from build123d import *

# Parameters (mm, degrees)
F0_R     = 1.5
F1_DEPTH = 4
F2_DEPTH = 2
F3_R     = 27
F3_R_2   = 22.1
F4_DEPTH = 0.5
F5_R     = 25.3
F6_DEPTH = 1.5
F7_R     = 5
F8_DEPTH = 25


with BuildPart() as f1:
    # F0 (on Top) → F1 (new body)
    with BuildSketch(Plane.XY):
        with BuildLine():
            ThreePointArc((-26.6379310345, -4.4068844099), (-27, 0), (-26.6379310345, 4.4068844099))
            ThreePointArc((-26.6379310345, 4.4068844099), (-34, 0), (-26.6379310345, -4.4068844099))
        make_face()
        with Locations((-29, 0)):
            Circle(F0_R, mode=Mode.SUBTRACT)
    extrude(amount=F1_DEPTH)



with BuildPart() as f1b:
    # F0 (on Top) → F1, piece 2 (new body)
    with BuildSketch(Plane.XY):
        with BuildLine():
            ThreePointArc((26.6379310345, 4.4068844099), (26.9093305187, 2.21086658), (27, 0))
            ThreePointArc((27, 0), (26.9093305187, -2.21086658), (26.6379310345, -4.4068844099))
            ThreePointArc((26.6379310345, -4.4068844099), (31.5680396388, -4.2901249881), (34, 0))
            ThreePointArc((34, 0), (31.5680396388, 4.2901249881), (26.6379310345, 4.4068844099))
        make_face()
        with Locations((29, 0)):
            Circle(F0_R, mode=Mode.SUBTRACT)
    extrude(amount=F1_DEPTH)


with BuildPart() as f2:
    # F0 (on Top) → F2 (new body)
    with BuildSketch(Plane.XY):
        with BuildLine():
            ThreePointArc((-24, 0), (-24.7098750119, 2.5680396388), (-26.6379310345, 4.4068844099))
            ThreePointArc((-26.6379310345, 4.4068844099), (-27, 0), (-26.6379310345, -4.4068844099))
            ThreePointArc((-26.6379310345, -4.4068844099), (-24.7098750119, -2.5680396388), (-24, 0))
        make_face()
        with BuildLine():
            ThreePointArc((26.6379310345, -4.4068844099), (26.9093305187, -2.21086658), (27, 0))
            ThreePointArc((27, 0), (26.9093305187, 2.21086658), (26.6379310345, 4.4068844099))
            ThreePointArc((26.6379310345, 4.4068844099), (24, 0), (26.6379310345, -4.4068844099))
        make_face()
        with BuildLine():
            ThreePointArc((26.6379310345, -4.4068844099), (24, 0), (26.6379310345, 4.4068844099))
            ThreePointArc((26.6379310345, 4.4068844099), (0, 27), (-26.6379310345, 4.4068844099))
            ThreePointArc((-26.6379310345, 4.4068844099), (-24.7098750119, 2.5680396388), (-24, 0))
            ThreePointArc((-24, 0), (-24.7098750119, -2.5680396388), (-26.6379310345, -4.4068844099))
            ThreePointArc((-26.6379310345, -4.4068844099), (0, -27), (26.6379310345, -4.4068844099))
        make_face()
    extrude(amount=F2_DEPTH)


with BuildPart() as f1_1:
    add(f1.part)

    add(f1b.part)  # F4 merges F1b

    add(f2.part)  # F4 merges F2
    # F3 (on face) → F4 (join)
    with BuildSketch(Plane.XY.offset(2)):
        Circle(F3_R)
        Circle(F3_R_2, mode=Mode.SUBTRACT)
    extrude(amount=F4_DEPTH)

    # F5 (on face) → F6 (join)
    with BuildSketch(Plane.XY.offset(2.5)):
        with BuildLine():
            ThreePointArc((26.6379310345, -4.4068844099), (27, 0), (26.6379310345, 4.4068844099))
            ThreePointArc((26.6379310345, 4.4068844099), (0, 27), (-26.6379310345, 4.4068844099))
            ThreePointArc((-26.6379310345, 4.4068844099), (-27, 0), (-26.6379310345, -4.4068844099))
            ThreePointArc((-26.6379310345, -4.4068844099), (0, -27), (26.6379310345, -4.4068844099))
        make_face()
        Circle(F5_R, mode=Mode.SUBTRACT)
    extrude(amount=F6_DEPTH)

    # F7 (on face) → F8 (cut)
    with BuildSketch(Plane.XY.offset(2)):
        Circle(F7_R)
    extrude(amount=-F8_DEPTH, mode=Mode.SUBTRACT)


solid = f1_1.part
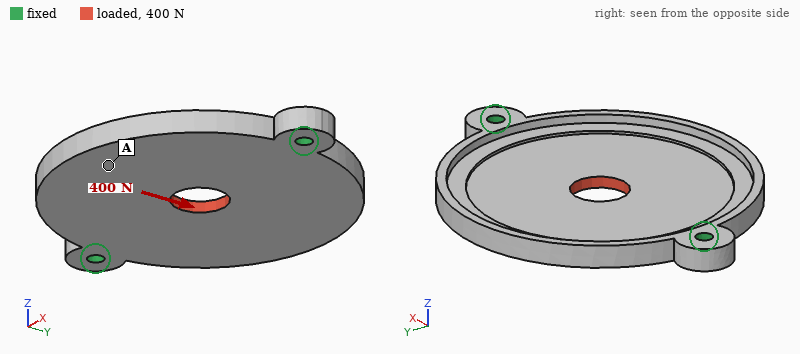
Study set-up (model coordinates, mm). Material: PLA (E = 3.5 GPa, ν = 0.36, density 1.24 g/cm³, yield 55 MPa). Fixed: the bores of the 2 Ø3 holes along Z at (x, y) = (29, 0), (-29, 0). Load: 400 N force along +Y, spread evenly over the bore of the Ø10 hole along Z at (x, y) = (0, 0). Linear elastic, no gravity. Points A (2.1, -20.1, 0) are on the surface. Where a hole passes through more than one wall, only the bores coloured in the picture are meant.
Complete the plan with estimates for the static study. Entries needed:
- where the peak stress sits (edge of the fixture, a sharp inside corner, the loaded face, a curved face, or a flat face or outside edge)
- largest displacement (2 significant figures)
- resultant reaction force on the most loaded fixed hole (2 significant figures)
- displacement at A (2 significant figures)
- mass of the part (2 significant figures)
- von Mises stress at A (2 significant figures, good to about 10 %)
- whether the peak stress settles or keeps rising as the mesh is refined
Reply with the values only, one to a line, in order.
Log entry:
edge of the fixture
0.29 mm
200 N
0.21 mm
7.0 g
3.3 MPa
keeps rising
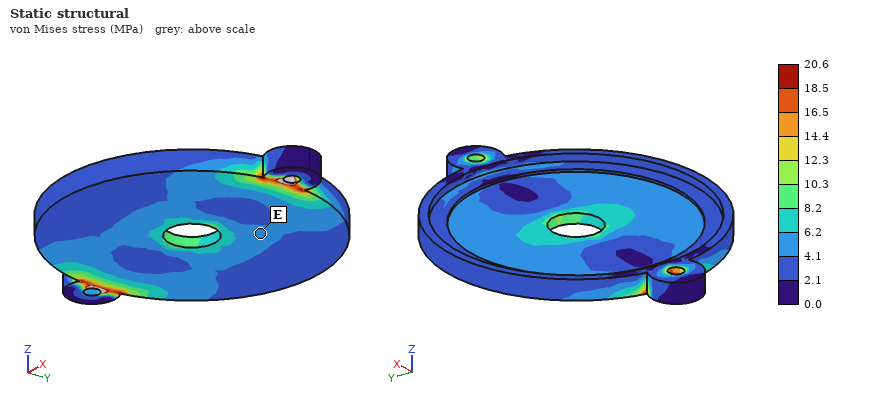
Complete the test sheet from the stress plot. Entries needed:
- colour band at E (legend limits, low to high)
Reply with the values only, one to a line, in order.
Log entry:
4.1 to 6.2 MPa
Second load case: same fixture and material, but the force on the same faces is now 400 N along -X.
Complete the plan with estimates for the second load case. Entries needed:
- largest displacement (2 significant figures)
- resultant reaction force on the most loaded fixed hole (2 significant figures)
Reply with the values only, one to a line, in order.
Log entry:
53 µm
200 N
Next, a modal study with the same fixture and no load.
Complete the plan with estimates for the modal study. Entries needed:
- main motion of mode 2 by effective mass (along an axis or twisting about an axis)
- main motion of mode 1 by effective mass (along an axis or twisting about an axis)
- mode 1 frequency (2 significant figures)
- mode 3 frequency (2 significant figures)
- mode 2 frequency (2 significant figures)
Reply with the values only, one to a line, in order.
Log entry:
along Z
twisting about X
720 Hz
2100 Hz
870 Hz
